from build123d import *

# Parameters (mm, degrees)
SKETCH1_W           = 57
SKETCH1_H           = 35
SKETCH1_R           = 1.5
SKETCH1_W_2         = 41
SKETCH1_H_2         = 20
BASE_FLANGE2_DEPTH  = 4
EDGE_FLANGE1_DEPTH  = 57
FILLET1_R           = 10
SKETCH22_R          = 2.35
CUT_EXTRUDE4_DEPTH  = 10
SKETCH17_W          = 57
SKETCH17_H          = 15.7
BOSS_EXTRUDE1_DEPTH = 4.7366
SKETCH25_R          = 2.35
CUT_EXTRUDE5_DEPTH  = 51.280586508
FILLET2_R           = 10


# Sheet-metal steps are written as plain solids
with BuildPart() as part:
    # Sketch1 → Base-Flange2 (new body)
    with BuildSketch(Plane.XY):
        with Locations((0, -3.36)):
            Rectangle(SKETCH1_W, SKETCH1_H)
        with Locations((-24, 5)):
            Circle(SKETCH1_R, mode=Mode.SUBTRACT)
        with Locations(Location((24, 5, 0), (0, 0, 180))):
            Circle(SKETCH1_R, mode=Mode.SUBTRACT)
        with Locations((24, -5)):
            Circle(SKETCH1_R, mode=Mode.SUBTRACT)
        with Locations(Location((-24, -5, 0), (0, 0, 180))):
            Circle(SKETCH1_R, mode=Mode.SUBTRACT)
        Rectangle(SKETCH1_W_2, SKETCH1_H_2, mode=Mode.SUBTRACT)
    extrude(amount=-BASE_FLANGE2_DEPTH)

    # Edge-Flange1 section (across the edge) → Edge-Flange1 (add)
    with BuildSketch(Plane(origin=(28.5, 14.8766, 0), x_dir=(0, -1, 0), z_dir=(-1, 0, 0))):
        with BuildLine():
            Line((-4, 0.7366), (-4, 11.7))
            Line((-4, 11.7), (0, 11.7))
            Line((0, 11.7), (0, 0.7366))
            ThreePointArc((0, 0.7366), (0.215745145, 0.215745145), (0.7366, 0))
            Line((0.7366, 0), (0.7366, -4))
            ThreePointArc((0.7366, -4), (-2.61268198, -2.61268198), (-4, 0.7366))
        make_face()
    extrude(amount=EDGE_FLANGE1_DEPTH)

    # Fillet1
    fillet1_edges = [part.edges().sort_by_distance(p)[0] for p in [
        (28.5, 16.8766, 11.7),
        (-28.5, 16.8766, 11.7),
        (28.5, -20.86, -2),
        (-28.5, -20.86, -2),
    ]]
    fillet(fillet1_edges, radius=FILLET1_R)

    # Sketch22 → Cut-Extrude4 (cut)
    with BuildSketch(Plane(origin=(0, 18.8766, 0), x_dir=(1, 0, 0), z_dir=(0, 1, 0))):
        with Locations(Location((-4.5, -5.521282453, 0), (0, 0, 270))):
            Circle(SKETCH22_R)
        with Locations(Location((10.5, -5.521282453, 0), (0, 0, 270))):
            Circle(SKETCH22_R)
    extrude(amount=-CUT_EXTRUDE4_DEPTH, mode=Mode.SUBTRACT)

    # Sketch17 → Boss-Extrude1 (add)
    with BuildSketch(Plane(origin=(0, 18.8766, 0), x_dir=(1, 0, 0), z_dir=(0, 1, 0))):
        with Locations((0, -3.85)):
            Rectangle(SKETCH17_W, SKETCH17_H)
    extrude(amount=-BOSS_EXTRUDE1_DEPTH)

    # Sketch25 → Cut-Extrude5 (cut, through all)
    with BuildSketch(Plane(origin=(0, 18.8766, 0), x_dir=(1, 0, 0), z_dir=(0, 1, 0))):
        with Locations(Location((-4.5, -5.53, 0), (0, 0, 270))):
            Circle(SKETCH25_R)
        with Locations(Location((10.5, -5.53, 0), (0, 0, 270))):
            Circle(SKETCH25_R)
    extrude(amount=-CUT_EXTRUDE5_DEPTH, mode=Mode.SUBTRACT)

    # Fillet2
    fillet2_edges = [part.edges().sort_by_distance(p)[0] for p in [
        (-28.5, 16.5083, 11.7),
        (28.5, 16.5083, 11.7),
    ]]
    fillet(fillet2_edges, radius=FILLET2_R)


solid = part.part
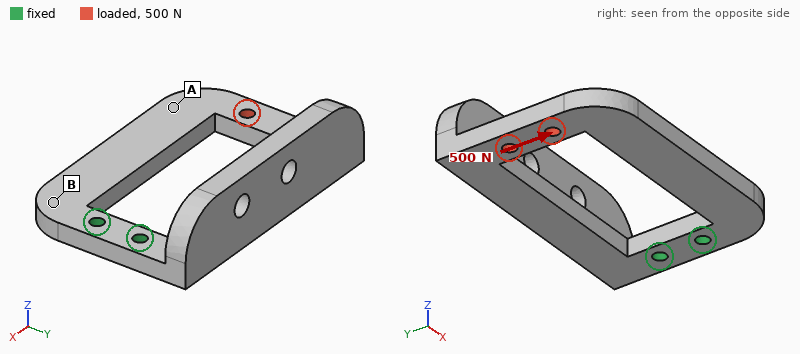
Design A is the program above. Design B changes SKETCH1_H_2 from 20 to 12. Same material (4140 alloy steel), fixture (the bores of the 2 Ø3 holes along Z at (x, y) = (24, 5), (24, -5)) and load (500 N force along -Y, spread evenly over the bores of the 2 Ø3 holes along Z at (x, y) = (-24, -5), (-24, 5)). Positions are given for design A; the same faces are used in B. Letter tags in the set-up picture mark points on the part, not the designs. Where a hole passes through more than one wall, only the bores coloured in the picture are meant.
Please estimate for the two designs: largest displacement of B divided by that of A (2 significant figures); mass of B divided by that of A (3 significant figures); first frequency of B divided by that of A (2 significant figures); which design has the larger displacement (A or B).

0.63
1.16
1.2
A
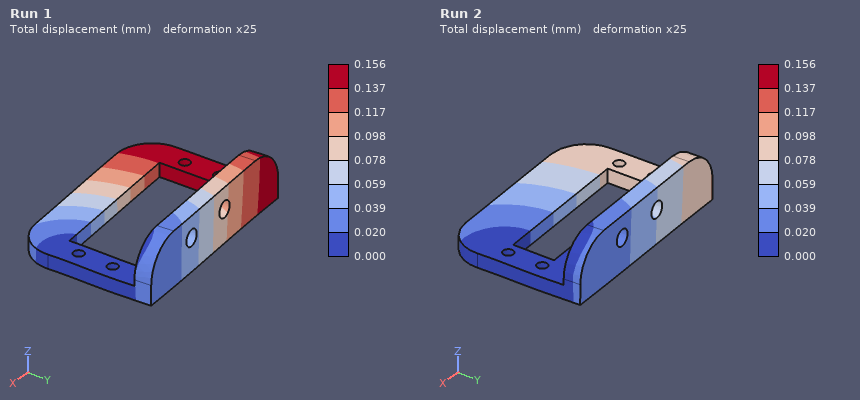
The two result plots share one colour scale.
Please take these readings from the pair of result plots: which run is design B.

Run 2
